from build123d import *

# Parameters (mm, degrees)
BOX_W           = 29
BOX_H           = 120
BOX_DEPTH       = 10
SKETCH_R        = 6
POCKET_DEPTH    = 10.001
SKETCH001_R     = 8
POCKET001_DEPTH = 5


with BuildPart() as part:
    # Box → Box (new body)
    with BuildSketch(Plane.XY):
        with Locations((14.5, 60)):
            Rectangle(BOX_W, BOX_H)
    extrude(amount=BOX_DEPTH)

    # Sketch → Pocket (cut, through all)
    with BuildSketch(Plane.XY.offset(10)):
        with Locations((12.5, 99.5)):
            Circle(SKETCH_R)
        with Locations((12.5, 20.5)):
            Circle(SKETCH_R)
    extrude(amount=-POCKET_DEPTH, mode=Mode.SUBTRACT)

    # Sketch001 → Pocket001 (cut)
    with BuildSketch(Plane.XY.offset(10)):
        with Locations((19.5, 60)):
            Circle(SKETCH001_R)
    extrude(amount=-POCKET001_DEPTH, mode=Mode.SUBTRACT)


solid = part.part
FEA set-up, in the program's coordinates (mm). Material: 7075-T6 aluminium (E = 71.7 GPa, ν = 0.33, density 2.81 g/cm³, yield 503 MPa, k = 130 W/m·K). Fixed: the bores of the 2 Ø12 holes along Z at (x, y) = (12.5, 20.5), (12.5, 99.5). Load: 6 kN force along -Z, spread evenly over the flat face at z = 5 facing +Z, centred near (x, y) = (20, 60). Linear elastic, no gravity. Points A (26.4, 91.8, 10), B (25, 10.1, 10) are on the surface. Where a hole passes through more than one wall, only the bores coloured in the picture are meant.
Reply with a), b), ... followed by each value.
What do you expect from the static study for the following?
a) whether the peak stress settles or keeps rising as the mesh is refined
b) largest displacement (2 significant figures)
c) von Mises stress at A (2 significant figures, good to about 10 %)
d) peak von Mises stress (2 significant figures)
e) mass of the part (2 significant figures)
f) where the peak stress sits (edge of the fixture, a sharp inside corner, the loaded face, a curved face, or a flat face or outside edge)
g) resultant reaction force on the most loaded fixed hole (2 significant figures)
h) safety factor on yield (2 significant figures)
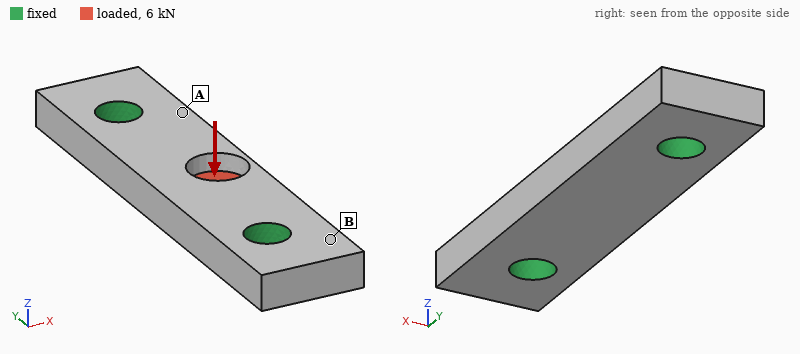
a) settles
b) 0.14 mm
c) 78 MPa
d) 370 MPa
e) 89 g
f) a curved face
g) 3.4 kN
h) 1.4
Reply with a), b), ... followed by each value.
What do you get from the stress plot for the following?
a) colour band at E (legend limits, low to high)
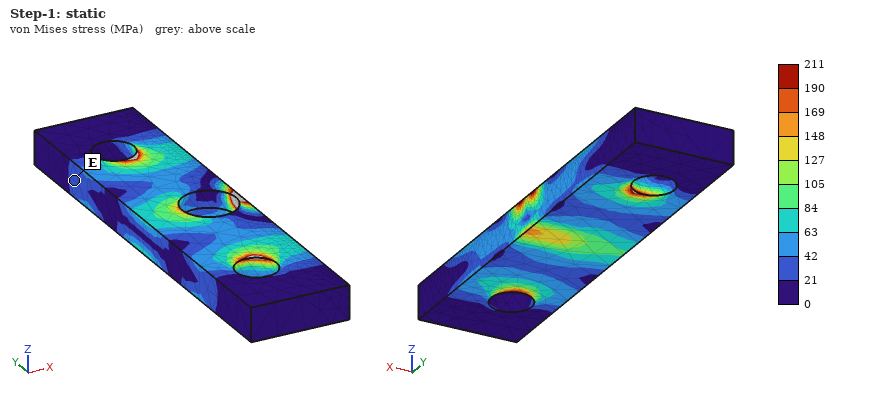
a) 21 to 42 MPa
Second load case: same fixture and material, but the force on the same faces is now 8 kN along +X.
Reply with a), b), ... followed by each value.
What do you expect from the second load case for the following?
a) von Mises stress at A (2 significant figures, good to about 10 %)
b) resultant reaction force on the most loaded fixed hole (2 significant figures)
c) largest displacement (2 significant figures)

a) 21 MPa
b) 4.0 kN
c) 47 µm
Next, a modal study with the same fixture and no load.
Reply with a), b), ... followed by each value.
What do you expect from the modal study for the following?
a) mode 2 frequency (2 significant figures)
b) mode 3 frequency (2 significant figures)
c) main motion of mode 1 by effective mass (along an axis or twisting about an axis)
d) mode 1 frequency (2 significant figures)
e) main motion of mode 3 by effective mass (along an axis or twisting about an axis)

a) 13 kHz
b) 15 kHz
c) along Z
d) 8900 Hz
e) along X
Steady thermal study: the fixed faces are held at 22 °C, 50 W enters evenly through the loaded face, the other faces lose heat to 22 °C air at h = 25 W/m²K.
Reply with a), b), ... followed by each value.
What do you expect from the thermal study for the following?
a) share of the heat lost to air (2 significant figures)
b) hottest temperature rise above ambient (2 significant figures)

a) 3.5 %
b) 33 K
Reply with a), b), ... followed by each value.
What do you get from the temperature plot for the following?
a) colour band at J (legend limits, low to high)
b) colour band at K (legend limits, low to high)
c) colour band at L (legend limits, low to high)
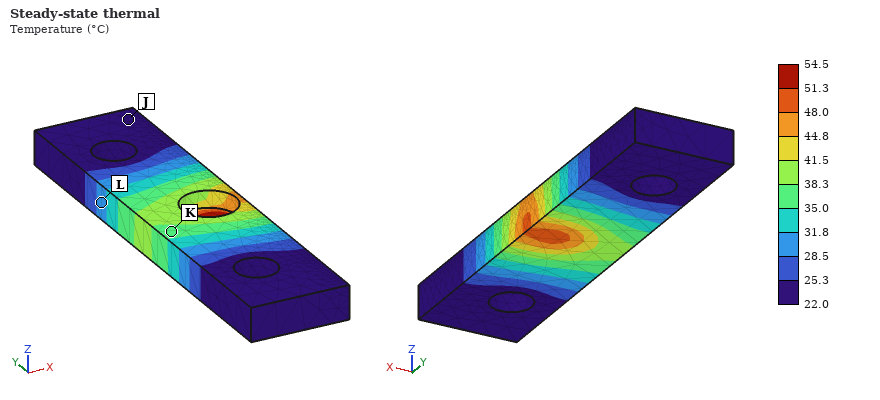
a) 22.0 to 25.3 °C
b) 35.0 to 38.3 °C
c) 28.5 to 31.8 °C
